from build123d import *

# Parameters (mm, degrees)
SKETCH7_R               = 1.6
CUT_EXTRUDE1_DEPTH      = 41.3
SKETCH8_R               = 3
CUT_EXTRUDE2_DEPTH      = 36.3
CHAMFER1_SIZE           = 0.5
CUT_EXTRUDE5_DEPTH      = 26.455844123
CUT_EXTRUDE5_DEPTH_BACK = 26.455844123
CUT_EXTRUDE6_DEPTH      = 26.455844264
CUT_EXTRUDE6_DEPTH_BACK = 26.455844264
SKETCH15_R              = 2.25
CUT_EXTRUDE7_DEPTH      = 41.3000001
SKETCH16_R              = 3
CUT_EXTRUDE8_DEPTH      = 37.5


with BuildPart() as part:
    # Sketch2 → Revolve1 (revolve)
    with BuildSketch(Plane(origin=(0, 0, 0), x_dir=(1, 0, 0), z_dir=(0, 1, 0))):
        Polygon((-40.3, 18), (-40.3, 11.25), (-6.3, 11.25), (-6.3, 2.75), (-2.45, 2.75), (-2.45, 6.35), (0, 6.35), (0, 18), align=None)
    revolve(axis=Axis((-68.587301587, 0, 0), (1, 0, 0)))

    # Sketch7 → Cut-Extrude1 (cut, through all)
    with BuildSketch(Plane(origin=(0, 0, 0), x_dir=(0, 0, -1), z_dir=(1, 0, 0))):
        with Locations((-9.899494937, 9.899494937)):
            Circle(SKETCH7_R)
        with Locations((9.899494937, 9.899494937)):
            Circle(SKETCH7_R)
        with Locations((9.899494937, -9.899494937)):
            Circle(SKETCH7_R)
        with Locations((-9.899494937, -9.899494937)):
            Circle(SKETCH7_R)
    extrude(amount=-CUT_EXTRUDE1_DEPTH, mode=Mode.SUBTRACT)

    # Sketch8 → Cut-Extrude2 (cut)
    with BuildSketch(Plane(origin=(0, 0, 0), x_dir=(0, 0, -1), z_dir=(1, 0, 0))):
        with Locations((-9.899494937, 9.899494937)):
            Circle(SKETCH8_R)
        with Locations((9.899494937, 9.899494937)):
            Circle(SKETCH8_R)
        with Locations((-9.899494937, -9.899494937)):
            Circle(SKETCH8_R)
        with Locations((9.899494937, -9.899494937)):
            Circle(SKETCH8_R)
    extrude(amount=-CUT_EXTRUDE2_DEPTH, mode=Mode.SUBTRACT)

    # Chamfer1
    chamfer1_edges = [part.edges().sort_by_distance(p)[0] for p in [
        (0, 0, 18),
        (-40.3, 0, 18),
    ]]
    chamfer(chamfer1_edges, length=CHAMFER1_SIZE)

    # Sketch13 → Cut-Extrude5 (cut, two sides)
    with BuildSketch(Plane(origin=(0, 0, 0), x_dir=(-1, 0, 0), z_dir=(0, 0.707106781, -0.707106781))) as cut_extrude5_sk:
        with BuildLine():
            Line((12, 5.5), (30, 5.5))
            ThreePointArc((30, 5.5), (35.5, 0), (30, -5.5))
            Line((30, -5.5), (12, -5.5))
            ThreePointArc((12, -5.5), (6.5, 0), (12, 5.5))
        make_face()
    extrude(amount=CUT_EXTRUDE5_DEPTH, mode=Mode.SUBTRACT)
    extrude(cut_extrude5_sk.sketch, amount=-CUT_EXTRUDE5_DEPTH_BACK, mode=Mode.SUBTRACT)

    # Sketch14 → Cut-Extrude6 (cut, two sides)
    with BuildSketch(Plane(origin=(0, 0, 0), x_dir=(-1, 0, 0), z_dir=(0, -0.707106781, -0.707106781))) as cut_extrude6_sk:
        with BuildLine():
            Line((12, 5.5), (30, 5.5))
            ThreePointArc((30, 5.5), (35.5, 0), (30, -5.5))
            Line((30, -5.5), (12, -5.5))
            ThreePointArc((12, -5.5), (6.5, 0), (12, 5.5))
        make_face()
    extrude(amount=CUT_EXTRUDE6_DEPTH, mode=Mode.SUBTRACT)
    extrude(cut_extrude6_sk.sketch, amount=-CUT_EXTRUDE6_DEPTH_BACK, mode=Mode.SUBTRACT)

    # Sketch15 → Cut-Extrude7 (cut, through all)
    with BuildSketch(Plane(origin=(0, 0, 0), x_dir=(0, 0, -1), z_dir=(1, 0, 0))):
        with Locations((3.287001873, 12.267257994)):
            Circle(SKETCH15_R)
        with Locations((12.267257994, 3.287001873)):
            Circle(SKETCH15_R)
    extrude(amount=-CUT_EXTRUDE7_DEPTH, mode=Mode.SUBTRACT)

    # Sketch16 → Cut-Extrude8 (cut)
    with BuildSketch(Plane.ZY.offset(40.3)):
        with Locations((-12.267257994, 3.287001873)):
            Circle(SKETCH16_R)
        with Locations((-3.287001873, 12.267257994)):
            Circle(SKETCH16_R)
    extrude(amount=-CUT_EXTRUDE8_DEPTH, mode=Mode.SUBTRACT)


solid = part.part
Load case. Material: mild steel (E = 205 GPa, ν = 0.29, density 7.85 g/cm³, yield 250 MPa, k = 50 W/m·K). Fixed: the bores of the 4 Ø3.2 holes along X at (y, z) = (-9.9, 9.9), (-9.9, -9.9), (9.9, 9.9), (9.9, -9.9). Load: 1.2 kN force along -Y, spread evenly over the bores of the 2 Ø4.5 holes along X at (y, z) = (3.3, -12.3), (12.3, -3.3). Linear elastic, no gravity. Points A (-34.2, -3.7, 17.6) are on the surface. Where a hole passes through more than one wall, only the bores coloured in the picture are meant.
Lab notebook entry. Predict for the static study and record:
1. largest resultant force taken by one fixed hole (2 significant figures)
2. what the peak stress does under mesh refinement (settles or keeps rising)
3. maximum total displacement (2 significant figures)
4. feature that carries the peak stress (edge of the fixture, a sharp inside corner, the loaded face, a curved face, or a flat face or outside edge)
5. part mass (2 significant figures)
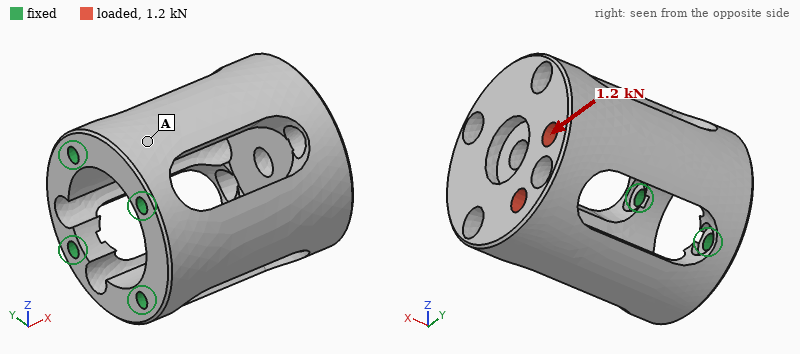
1.1 kN
keeps rising
31 µm
edge of the fixture
130 g
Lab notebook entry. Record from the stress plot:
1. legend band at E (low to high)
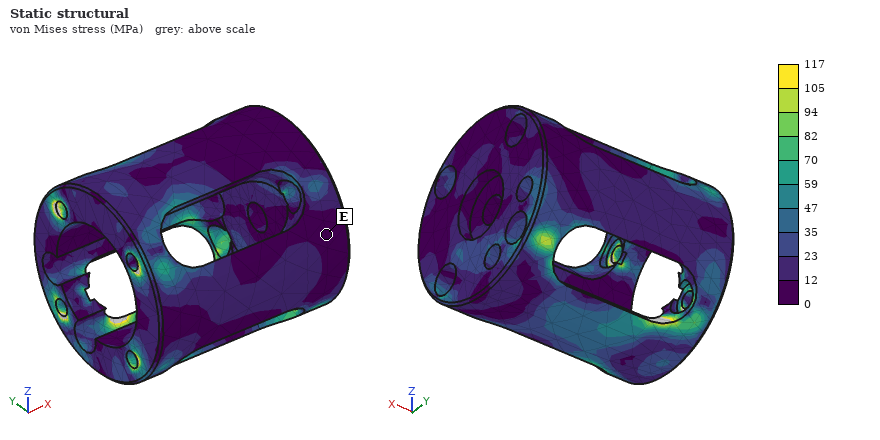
0 to 12 MPa
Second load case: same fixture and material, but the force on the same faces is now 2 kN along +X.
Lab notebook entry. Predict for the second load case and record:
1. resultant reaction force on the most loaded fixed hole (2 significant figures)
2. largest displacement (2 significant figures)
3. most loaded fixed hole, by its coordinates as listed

870 N
14 µm
(9.9, -9.9)
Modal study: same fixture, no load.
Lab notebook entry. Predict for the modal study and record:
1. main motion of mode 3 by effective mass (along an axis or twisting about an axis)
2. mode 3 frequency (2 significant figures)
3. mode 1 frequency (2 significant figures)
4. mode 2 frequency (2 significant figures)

twisting about X
9100 Hz
4500 Hz
4600 Hz
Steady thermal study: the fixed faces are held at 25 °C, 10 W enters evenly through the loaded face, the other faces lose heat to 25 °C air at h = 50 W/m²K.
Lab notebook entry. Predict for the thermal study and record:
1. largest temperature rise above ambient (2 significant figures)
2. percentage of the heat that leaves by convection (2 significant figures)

30 K
47 %
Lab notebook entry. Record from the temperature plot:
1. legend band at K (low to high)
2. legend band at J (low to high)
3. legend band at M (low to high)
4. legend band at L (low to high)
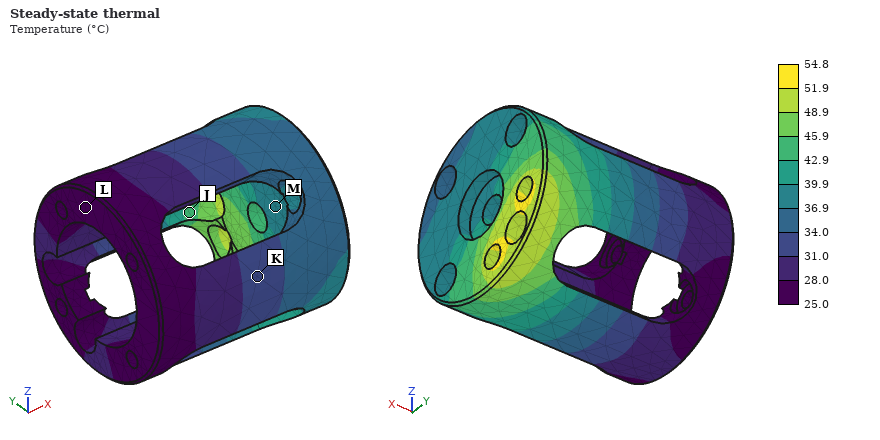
31.0 to 34.0 °C
42.9 to 45.9 °C
36.9 to 39.9 °C
25.0 to 28.0 °C
